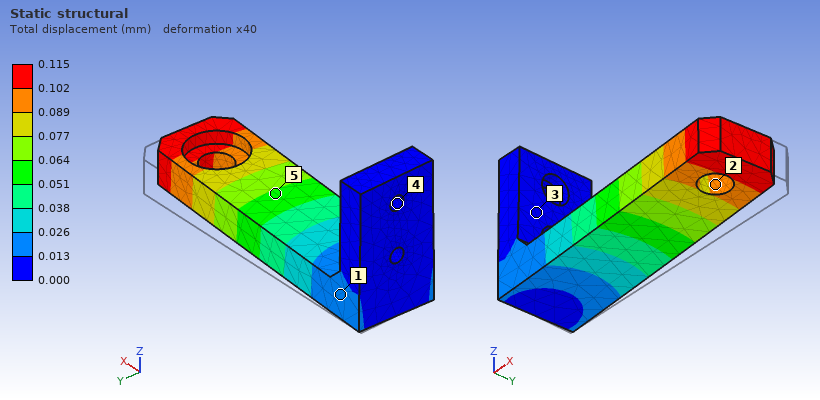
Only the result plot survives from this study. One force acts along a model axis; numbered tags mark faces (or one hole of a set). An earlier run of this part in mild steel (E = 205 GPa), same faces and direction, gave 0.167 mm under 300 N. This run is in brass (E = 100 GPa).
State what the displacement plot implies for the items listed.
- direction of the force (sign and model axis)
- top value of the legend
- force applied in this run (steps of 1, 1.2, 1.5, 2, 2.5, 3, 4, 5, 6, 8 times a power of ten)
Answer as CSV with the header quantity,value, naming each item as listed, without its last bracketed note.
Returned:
quantity,value
direction of the force,-Y
top value of the legend,0.115 mm
force applied in this run,100 N
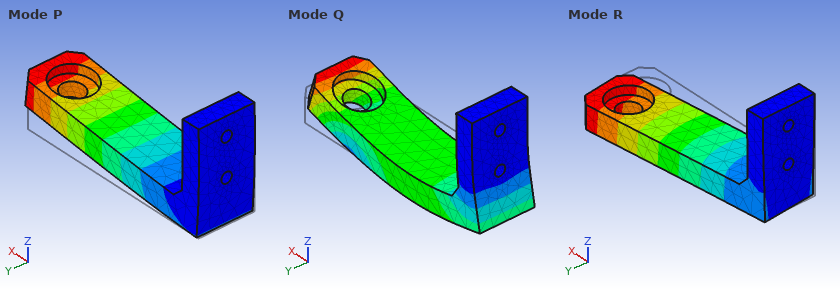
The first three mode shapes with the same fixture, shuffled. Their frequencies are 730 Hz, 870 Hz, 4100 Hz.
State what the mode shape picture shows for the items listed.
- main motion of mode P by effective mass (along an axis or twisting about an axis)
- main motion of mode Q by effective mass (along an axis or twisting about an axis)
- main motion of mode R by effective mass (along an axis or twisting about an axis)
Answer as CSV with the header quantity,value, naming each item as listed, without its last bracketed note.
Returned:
quantity,value
main motion of mode P by effective mass,along Z
main motion of mode Q by effective mass,along X
main motion of mode R by effective mass,along Y
